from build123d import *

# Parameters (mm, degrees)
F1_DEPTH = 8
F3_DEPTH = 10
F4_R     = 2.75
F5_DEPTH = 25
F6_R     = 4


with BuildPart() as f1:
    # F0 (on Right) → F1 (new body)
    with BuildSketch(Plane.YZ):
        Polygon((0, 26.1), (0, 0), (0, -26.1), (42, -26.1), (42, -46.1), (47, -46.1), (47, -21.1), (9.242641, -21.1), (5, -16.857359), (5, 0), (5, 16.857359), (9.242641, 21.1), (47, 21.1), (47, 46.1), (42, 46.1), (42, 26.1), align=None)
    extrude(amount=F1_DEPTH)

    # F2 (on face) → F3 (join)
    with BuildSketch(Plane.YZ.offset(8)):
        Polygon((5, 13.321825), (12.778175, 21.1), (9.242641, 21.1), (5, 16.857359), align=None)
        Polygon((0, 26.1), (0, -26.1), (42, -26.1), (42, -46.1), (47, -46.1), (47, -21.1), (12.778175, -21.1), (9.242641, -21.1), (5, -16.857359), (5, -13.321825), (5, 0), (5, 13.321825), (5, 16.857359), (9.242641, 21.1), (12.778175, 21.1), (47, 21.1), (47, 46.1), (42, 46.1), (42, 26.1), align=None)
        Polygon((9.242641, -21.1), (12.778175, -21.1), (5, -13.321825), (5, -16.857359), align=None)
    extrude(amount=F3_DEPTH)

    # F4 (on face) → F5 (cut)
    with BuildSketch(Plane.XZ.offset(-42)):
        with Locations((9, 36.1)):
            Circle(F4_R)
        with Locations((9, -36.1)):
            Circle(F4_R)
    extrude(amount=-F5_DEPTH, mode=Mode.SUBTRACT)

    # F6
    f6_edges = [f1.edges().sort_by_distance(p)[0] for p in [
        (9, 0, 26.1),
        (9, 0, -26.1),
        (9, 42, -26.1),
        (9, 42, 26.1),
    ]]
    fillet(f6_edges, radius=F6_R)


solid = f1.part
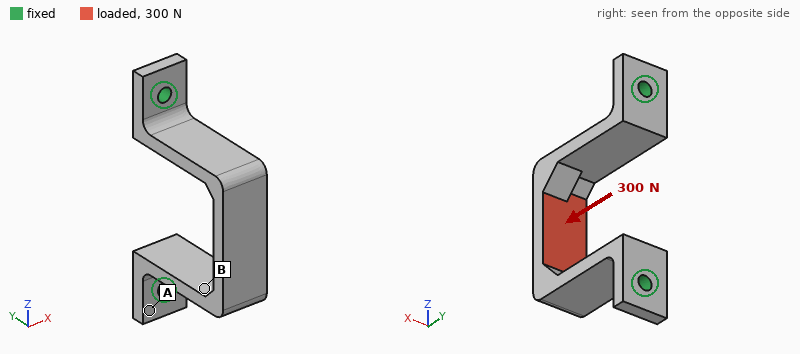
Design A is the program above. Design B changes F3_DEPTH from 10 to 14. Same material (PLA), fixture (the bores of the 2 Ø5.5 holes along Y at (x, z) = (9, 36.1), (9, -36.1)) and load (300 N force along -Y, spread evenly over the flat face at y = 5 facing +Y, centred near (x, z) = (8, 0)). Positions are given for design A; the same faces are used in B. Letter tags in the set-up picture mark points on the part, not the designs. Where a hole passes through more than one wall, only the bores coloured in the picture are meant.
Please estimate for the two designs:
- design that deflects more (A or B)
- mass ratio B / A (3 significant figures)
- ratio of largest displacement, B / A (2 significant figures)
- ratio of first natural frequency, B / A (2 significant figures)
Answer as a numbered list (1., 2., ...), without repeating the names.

1. A
2. 1.23
3. 0.79
4. 0.99
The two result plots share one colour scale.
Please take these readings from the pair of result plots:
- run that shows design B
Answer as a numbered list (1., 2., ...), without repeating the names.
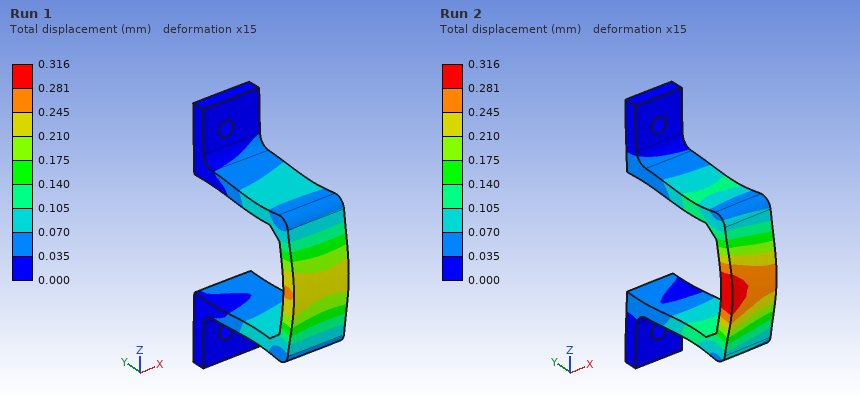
1. Run 1
